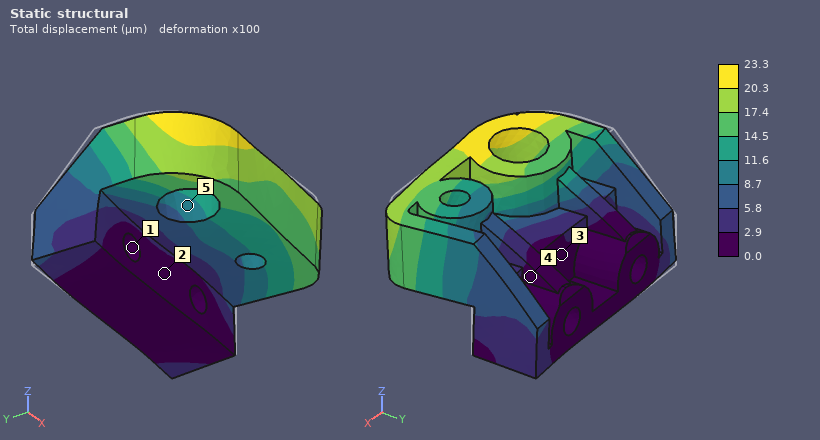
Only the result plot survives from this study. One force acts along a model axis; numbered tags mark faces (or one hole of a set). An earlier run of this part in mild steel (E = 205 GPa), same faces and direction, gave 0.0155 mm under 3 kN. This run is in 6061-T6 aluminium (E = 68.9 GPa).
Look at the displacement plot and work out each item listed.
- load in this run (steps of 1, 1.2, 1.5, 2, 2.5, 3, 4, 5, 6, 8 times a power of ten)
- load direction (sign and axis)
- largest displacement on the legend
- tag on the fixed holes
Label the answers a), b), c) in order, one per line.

a) 1.5 kN
b) +X
c) 23.3 µm
d) 1
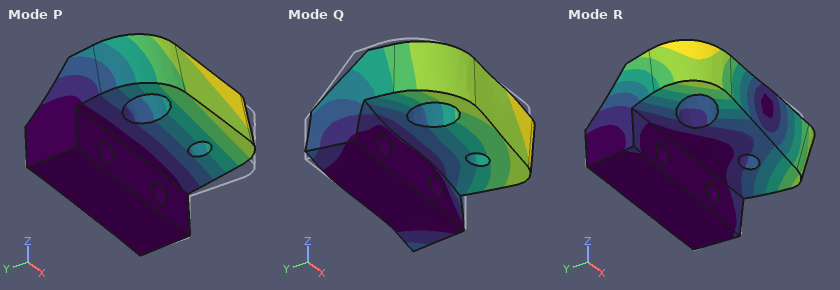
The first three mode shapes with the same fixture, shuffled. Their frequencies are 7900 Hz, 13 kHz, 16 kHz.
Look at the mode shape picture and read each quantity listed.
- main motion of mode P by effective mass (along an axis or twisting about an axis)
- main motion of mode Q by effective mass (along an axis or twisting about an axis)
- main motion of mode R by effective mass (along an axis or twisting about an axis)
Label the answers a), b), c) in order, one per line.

a) along Z
b) along X
c) twisting about Y
